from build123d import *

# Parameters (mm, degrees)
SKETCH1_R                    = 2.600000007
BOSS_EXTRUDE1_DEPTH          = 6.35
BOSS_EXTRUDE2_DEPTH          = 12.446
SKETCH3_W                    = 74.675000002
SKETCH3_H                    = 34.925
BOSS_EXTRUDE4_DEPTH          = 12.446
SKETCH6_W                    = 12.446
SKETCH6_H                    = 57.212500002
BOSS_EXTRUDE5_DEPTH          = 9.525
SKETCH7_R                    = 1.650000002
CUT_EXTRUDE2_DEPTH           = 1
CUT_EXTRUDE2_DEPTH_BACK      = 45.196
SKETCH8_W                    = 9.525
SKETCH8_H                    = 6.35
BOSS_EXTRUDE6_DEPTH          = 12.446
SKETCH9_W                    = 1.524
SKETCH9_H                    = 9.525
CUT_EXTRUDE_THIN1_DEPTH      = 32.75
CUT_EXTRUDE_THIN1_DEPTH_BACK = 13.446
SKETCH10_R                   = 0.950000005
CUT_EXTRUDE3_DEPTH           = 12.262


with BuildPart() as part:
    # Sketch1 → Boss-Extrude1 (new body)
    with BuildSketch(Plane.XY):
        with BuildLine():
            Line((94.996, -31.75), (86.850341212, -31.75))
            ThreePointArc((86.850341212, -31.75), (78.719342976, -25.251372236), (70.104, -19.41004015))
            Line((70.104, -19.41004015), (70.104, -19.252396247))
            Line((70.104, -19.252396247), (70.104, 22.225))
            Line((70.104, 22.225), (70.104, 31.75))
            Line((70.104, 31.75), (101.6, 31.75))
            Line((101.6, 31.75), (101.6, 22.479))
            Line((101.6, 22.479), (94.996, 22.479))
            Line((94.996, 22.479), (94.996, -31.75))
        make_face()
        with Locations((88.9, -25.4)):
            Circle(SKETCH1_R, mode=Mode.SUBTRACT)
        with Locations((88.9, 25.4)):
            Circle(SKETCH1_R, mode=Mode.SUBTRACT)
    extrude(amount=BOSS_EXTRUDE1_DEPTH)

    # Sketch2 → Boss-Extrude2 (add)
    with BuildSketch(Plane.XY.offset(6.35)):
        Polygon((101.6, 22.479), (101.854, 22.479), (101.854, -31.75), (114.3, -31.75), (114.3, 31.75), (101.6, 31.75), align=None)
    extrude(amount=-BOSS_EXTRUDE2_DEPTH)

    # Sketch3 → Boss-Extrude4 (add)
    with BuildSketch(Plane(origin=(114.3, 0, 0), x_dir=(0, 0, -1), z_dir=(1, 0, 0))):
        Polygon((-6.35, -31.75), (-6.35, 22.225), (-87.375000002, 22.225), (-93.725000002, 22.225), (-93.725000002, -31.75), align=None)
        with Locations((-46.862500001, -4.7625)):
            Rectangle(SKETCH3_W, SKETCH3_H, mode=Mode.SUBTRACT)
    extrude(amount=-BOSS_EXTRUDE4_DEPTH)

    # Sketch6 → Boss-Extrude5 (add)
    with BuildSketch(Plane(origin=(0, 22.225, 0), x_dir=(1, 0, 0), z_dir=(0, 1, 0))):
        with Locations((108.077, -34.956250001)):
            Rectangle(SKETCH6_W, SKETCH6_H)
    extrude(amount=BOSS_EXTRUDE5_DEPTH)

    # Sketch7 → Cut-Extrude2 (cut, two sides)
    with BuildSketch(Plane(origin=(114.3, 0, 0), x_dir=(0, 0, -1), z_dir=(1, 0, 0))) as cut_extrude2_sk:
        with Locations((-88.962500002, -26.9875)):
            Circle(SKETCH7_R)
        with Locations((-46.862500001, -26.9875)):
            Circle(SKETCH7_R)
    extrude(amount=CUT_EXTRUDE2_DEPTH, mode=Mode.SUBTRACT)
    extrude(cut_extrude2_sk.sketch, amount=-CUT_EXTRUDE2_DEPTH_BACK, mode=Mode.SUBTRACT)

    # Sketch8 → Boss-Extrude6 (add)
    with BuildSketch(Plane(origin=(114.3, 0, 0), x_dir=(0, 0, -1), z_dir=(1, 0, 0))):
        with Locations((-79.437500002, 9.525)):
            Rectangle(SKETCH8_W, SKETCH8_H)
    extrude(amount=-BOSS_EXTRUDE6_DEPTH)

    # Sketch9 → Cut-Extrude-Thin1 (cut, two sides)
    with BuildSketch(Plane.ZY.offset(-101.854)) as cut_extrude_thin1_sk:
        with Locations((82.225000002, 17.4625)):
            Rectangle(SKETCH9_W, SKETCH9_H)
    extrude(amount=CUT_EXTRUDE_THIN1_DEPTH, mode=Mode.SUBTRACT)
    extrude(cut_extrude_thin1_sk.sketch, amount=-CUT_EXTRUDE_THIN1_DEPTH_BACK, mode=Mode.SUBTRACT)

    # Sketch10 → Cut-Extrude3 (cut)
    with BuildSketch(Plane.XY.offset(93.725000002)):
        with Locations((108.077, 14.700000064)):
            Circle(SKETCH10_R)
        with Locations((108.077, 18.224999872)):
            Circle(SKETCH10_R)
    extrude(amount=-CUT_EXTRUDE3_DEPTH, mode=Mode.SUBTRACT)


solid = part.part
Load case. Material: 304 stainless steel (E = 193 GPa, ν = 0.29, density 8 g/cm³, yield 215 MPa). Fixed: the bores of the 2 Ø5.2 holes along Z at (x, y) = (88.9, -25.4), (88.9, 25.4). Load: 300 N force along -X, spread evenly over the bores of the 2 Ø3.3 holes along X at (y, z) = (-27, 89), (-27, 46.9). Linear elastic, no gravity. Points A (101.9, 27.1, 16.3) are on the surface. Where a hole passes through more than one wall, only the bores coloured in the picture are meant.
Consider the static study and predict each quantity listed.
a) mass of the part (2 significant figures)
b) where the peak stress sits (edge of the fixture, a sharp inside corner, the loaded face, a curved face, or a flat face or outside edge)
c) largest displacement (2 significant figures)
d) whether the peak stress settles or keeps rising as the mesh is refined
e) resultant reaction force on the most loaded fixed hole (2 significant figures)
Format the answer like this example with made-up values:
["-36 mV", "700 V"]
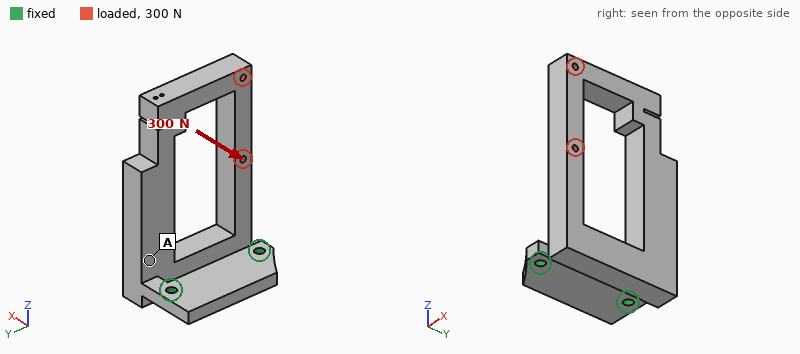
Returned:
["420 g", "a sharp inside corner", "0.88 mm", "keeps rising", "160 N"]
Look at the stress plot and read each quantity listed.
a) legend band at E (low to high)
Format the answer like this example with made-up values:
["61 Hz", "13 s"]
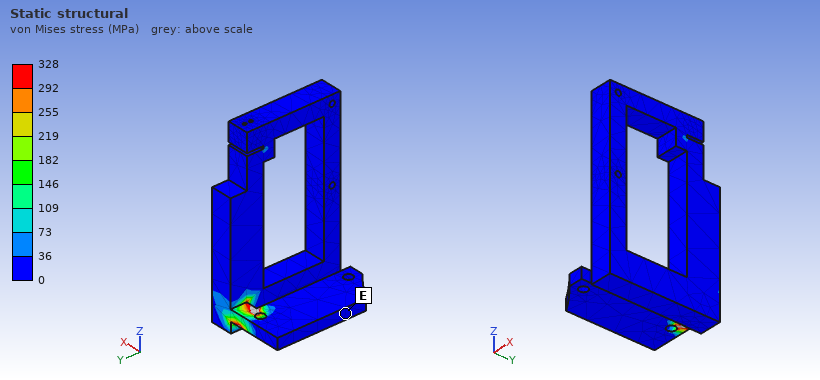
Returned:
["0 to 36 MPa"]
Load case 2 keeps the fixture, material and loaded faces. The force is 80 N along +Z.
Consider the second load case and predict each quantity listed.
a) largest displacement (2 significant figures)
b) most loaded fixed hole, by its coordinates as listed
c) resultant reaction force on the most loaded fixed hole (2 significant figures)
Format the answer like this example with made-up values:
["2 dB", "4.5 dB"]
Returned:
["0.15 mm", "(88.9, 25.4)", "75 N"]
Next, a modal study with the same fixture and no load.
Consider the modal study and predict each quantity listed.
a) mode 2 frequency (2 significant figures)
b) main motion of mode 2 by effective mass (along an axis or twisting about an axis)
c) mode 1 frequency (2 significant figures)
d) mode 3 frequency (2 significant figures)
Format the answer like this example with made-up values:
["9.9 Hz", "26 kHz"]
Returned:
["280 Hz", "along X", "260 Hz", "740 Hz"]
